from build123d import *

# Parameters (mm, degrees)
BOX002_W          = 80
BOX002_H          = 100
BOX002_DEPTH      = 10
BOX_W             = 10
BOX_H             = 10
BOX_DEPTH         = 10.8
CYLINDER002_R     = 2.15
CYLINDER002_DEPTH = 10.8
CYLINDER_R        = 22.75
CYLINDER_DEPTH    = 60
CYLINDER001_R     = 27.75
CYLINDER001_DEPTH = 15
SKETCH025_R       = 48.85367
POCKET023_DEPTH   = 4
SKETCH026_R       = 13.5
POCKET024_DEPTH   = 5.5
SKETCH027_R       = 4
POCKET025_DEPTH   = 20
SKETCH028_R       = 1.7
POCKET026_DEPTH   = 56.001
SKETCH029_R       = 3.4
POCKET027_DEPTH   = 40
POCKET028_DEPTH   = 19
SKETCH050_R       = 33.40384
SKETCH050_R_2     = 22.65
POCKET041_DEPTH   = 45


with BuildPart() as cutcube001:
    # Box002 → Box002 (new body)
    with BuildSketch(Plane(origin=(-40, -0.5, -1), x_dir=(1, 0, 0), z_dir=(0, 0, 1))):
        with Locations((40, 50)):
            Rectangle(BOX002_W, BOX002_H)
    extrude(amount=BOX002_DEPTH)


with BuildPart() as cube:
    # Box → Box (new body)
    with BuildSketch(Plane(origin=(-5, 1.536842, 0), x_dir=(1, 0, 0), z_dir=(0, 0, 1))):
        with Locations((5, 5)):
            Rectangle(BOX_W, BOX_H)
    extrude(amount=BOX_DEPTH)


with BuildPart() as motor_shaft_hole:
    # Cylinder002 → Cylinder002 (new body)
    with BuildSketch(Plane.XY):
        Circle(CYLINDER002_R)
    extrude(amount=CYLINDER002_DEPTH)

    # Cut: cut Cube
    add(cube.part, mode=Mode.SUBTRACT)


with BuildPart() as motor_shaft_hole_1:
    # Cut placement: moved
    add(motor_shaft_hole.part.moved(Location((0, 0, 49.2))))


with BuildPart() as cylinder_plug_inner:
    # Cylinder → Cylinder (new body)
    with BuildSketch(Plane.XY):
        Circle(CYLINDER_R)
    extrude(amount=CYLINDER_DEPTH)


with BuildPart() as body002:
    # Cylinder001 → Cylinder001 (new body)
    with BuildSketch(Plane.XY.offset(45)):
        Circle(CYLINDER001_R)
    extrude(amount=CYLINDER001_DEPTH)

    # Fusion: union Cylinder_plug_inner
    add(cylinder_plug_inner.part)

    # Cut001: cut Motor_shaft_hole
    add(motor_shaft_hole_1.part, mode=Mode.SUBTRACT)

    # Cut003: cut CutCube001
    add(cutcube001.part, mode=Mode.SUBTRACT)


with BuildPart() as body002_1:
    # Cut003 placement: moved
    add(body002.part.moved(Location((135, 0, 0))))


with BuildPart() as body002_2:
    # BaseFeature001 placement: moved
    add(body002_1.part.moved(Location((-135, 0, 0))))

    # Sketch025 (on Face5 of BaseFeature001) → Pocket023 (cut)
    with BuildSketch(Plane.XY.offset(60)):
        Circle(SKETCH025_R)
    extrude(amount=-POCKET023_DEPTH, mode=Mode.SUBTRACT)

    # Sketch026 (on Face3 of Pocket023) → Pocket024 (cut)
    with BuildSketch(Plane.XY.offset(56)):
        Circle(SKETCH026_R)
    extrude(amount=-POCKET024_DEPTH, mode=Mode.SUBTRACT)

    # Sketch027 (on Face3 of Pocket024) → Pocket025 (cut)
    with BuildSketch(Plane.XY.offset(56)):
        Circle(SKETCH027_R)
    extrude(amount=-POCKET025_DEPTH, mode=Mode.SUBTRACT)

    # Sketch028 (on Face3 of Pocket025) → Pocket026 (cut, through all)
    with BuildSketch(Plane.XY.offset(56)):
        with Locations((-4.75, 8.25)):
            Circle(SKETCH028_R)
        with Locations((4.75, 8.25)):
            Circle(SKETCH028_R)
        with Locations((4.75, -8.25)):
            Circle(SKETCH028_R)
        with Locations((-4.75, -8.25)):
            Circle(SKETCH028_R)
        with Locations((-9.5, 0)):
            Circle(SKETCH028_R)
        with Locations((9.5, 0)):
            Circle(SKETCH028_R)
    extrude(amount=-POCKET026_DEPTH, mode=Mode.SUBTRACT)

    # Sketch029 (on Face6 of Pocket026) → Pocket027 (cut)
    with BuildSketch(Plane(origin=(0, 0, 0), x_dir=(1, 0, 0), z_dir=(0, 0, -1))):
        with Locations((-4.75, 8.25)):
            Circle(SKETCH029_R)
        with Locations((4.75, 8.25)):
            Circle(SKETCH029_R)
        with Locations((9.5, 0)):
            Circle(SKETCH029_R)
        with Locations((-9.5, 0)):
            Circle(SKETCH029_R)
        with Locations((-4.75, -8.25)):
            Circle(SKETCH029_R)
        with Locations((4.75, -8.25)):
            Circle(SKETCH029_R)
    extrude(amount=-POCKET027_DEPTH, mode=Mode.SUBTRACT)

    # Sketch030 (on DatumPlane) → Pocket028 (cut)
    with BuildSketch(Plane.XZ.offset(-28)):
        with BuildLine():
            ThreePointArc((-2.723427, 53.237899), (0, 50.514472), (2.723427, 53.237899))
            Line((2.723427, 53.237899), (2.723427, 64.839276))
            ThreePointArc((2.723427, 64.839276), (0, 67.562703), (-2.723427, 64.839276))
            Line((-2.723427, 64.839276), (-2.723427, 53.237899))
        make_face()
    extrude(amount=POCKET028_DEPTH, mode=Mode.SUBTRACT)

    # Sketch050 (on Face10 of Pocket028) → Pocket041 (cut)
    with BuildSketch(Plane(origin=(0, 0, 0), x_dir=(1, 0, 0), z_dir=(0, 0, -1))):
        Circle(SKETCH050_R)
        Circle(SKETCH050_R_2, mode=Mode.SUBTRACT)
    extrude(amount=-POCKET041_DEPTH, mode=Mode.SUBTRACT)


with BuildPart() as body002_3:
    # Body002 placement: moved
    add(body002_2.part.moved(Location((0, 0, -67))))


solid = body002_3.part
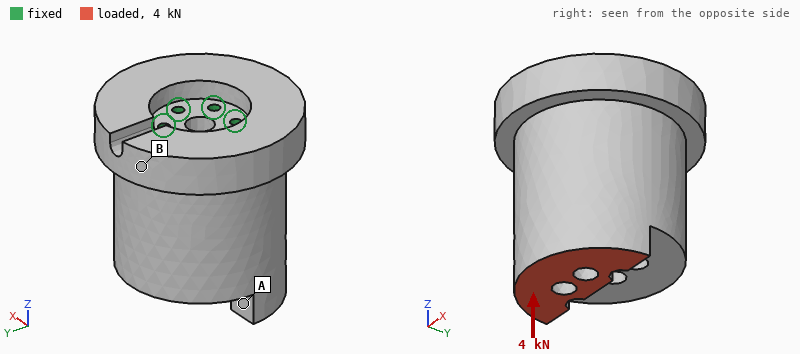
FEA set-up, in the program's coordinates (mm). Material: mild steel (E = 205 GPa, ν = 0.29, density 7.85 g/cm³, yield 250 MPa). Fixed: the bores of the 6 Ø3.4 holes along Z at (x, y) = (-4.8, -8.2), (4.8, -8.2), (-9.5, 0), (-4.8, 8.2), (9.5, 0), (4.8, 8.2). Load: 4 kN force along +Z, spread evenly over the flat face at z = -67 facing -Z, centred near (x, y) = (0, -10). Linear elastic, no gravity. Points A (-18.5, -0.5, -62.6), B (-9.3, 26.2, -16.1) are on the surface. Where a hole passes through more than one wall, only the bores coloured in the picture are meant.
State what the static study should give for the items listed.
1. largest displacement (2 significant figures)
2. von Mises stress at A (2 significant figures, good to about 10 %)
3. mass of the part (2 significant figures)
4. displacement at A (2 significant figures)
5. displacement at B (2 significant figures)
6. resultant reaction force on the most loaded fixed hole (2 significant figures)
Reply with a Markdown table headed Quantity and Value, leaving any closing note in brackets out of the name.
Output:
| Quantity | Value |
|---|---|
| largest displacement | 3.9 µm |
| von Mises stress at A | 6.5 MPa |
| mass of the part | 620 g |
| displacement at A | 2.5 µm |
| displacement at B | 0.70 µm |
| resultant reaction force on the most loaded fixed hole | 1.5 kN |
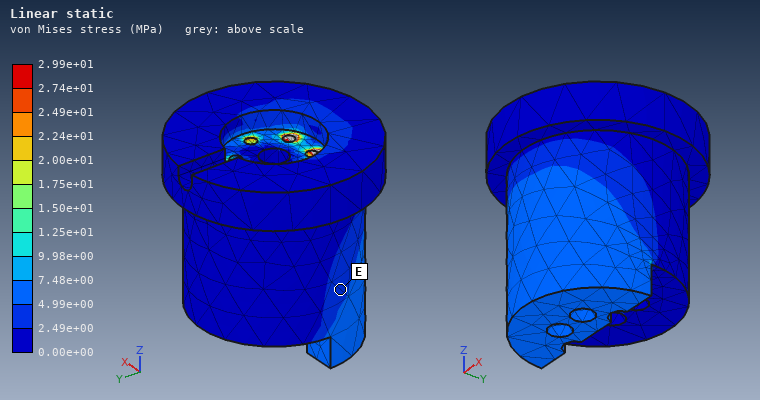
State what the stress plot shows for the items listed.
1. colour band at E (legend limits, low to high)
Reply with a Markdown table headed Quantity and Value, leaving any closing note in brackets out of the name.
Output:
| Quantity | Value |
|---|---|
| colour band at E | 2.49e+00 to 4.99e+00 MPa |
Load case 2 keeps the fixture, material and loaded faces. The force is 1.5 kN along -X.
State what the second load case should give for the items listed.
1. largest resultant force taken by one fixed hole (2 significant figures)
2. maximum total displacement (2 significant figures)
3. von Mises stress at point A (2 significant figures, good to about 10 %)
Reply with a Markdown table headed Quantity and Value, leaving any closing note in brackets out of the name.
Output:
| Quantity | Value |
|---|---|
| largest resultant force taken by one fixed hole | 1.5 kN |
| maximum total displacement | 6.3 µm |
| von Mises stress at point A | 4.3 MPa |
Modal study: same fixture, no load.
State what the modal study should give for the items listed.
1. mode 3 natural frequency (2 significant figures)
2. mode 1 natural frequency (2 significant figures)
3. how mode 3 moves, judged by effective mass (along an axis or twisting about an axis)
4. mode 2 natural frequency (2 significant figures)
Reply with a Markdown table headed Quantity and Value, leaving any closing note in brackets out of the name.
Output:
| Quantity | Value |
|---|---|
| mode 3 natural frequency | 14 kHz |
| mode 1 natural frequency | 7200 Hz |
| how mode 3 moves, judged by effective mass | twisting about Z |
| mode 2 natural frequency | 7200 Hz |
